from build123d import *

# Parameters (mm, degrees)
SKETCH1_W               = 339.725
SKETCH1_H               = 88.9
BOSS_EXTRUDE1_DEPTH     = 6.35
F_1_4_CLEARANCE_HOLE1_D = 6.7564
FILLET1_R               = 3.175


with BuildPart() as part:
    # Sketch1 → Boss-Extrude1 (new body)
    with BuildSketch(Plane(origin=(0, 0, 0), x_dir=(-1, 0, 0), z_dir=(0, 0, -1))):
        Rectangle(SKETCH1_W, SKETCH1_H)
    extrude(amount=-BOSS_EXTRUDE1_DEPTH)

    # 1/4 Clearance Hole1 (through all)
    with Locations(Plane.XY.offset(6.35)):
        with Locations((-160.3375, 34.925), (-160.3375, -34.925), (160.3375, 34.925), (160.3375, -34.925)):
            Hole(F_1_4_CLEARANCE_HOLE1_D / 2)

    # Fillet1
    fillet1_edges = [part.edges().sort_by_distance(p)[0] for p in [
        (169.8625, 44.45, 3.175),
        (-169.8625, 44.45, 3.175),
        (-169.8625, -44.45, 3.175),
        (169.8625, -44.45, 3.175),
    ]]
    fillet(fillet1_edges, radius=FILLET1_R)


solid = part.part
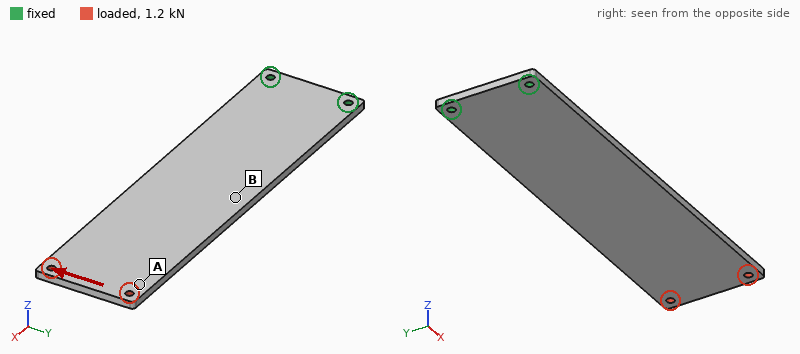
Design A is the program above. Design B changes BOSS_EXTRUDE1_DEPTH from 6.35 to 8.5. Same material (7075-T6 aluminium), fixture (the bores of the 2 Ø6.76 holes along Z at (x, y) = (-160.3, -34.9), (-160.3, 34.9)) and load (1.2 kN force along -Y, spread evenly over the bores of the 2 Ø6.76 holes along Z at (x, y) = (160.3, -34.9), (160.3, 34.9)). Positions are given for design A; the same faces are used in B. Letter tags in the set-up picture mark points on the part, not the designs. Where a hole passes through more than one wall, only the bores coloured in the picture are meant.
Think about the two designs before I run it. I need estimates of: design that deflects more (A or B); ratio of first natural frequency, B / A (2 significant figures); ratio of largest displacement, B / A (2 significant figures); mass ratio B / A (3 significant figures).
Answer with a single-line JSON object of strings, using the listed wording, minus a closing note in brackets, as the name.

{"design that deflects more": "A", "ratio of first natural frequency, B / A": "1.3", "ratio of largest displacement, B / A": "0.75", "mass ratio B / A": "1.34"}
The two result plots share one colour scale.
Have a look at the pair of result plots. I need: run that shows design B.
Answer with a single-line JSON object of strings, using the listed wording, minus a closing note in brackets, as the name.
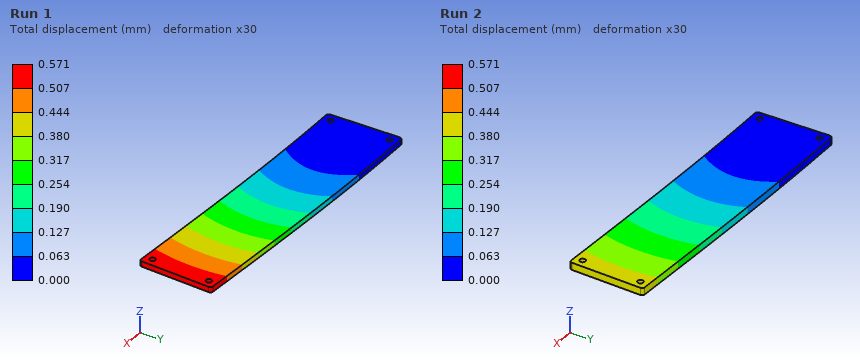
{"run that shows design B": "Run 2"}
